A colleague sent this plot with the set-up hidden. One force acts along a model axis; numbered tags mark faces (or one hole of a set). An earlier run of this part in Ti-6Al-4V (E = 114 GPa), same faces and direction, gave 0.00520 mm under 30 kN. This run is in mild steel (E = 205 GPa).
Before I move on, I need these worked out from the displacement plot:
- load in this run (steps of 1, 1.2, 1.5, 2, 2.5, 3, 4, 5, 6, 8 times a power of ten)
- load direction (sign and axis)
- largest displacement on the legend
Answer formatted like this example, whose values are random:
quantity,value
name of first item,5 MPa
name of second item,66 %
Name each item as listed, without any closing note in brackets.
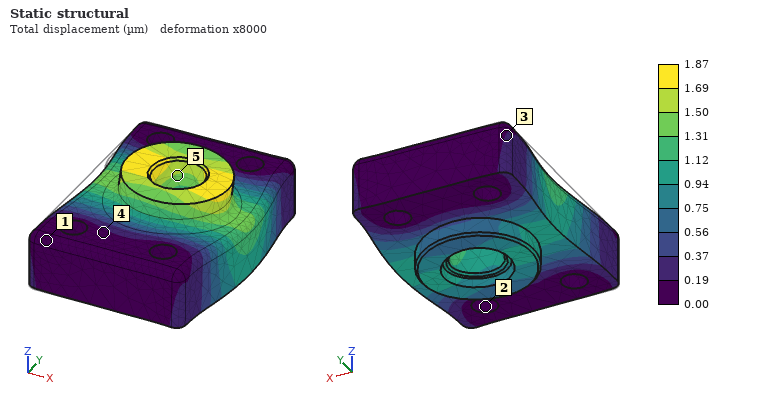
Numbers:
quantity,value
load in this run,20 kN
load direction,+X
largest displacement on the legend,1.87 µm
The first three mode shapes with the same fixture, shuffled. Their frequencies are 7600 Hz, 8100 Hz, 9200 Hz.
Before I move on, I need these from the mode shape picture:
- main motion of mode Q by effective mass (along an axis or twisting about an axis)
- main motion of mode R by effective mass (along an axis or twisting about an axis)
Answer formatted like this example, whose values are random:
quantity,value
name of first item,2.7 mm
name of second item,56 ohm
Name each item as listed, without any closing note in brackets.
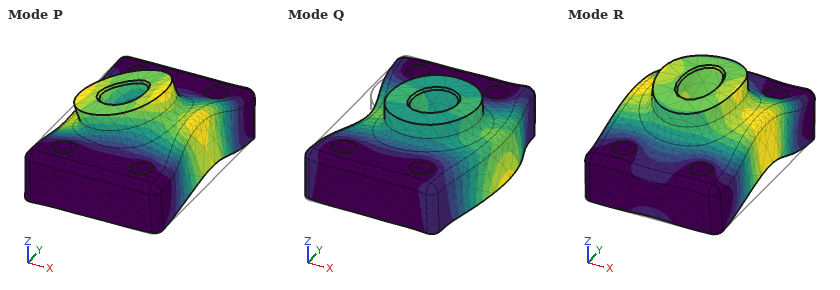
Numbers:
quantity,value
main motion of mode Q by effective mass,along X
main motion of mode R by effective mass,along Z
